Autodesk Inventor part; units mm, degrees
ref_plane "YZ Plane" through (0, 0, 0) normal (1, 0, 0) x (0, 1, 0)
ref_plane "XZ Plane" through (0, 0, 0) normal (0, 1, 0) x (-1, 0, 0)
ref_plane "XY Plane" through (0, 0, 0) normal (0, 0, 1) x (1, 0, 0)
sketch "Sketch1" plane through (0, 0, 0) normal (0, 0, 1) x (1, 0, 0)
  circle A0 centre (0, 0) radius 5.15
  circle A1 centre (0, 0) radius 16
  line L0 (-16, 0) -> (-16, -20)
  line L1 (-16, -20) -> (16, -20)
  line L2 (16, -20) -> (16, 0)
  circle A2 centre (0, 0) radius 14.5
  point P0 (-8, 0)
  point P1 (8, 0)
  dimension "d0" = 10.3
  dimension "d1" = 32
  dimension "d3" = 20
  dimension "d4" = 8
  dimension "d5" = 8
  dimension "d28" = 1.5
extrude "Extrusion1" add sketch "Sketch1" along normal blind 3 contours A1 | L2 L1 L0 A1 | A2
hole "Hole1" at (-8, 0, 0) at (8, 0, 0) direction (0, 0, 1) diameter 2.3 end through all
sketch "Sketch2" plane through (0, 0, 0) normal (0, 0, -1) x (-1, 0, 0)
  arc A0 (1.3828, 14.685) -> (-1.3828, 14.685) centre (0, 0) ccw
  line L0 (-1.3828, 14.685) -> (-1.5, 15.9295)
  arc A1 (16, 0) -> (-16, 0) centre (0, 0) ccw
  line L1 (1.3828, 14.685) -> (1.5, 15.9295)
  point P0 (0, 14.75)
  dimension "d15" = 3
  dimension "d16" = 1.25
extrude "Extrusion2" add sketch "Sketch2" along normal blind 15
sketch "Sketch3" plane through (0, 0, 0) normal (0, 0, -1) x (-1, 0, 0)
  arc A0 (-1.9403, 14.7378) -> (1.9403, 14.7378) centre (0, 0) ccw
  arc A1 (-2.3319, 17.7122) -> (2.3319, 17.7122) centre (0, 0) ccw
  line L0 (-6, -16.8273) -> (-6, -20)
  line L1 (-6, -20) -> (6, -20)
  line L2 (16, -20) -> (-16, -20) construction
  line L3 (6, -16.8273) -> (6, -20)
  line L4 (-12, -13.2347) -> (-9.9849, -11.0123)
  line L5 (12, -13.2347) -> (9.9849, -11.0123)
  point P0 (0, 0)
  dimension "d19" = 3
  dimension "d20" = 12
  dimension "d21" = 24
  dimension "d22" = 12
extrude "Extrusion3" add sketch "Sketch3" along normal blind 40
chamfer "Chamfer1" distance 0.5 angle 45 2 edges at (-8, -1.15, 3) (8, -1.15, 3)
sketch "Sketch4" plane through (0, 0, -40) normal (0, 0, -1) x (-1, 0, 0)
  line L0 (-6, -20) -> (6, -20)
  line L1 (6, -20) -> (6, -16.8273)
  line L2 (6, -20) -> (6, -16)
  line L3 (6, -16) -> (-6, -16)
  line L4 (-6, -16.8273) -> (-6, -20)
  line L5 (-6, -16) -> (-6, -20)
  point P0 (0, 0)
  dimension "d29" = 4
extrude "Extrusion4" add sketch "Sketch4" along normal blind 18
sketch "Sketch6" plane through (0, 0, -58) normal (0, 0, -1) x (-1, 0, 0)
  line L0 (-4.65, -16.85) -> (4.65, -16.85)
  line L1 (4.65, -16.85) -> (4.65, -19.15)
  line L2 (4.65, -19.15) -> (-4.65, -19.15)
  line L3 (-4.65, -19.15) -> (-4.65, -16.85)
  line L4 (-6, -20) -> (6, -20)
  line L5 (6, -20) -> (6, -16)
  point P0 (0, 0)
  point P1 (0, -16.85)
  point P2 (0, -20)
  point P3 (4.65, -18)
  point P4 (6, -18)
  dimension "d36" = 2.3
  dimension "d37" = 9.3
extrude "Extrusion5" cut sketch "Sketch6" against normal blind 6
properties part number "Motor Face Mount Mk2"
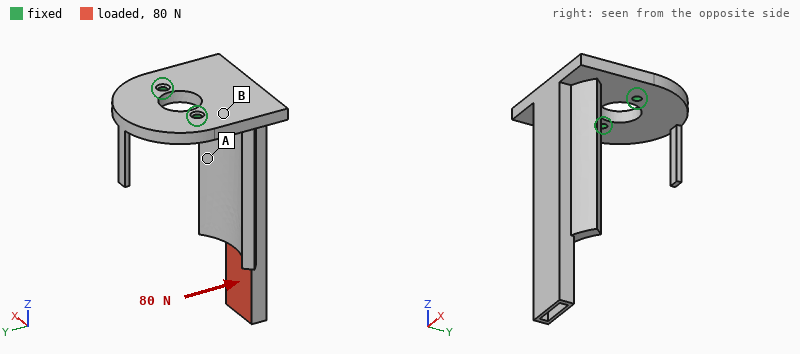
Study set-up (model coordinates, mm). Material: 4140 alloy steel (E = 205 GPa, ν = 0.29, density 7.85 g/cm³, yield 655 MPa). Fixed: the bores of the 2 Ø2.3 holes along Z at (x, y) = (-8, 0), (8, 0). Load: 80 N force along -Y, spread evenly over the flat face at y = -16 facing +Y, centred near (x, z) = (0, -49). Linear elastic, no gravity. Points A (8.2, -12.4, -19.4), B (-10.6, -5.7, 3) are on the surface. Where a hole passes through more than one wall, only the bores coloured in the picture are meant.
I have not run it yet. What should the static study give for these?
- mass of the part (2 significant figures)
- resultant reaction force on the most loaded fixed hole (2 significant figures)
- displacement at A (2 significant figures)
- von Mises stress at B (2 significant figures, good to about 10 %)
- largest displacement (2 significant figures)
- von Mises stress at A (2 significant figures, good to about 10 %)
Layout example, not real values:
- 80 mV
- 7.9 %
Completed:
- 61 g
- 42 N
- 0.12 mm
- 95 MPa
- 0.38 mm
- 17 MPa
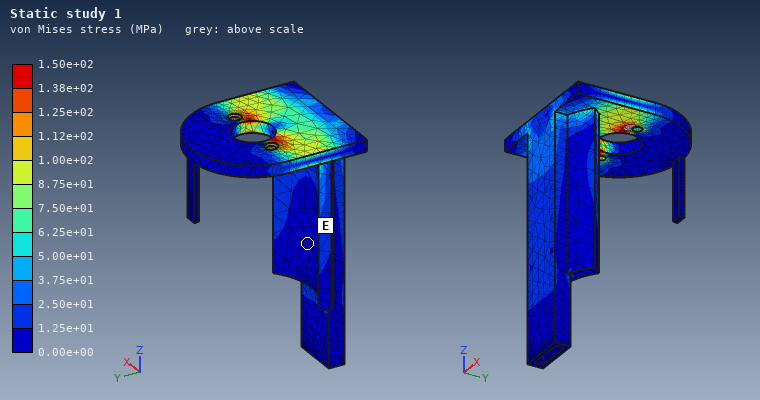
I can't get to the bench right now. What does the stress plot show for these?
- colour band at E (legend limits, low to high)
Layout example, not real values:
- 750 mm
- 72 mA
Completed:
- 0.00e+00 to 1.25e+01 MPa
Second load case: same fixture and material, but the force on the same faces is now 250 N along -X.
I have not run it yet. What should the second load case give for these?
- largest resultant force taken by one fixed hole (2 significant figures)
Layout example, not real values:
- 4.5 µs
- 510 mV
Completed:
- 640 N
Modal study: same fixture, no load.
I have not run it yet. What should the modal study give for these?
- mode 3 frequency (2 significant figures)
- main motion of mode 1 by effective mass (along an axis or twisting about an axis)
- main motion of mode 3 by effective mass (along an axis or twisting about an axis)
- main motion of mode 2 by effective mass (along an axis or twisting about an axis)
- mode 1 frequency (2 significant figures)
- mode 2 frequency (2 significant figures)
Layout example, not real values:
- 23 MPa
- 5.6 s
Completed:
- 3900 Hz
- along Y
- along Z
- along X
- 690 Hz
- 1600 Hz
